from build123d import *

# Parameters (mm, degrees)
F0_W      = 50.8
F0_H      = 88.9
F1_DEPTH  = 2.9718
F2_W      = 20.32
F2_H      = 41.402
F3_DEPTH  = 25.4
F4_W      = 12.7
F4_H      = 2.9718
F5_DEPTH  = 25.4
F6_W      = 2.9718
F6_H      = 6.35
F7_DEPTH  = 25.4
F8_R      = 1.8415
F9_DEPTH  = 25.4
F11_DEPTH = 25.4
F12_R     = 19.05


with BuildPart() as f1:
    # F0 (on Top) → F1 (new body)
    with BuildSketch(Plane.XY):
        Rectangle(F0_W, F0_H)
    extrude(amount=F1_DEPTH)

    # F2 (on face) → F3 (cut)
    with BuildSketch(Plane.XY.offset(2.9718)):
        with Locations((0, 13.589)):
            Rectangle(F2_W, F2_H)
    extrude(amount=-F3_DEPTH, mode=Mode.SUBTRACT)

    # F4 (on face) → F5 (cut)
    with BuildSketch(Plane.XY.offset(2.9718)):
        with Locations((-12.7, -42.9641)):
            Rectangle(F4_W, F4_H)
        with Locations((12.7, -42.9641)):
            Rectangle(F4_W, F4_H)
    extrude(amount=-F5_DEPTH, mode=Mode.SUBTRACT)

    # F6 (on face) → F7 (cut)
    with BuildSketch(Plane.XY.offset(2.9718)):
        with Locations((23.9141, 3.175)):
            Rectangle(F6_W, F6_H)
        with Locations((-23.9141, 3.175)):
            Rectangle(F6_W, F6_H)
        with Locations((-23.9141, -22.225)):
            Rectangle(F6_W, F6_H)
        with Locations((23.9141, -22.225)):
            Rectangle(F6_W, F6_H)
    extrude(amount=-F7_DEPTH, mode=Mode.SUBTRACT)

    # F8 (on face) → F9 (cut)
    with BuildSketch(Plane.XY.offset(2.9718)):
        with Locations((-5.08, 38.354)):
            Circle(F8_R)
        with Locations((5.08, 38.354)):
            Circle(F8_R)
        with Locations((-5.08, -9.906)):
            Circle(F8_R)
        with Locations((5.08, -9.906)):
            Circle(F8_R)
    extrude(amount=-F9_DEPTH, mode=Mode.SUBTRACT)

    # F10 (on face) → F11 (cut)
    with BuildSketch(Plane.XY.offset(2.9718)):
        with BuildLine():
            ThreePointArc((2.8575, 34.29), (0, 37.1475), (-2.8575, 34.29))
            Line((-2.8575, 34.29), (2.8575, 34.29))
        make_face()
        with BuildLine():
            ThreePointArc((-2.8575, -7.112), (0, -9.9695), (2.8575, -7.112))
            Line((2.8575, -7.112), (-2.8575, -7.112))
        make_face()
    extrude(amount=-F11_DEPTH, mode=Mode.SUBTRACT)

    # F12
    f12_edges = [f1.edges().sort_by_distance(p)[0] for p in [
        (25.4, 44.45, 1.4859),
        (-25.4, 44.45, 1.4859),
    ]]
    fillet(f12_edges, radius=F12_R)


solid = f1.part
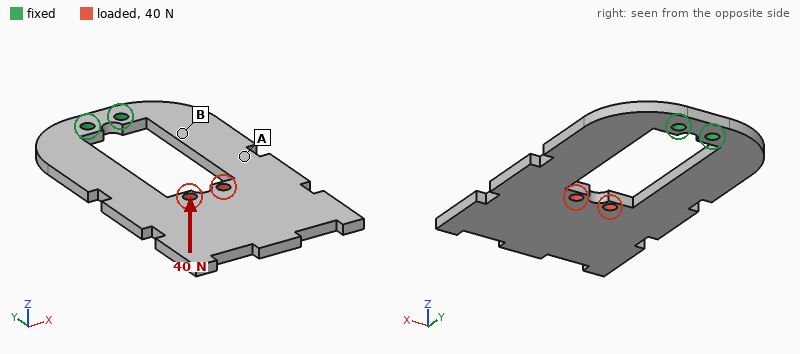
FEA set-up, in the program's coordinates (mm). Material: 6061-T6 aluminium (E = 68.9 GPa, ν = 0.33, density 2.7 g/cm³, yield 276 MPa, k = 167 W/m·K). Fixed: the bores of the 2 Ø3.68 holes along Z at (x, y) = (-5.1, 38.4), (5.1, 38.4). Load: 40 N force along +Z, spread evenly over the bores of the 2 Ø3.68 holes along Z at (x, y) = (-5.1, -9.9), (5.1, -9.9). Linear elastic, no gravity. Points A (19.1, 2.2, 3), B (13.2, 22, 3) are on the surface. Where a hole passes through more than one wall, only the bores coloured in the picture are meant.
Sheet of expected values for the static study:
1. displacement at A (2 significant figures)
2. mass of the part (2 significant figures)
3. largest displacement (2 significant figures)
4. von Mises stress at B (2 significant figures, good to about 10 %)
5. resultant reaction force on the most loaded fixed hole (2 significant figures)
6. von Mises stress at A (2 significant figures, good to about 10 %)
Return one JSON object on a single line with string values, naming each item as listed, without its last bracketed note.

{"displacement at A": "0.35 mm", "mass of the part": "26 g", "largest displacement": "1.0 mm", "von Mises stress at B": "30 MPa", "resultant reaction force on the most loaded fixed hole": "20 N", "von Mises stress at A": "14 MPa"}
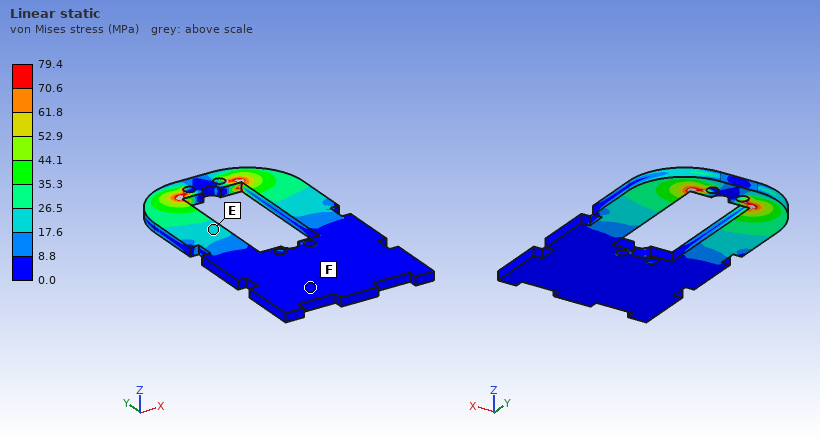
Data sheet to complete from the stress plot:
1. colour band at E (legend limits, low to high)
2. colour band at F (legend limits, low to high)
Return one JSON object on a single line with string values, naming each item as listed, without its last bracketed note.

{"colour band at E": "17.6 to 26.5 MPa", "colour band at F": "0.0 to 8.8 MPa"}
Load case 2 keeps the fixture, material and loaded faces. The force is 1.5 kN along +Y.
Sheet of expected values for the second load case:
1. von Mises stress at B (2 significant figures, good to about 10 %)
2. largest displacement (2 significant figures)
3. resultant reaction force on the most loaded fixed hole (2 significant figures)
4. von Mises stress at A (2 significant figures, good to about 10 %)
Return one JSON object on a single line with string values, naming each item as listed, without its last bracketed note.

{"von Mises stress at B": "35 MPa", "largest displacement": "46 µm", "resultant reaction force on the most loaded fixed hole": "800 N", "von Mises stress at A": "16 MPa"}
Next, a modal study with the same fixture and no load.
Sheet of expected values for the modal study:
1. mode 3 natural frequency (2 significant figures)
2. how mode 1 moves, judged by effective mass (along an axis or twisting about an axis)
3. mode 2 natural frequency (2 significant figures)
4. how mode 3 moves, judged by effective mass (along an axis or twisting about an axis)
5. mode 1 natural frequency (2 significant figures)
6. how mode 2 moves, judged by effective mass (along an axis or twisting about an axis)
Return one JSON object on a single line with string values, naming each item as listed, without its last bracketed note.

{"mode 3 natural frequency": "1200 Hz", "how mode 1 moves, judged by effective mass": "along Z", "mode 2 natural frequency": "830 Hz", "how mode 3 moves, judged by effective mass": "along X", "mode 1 natural frequency": "240 Hz", "how mode 2 moves, judged by effective mass": "twisting about Y"}
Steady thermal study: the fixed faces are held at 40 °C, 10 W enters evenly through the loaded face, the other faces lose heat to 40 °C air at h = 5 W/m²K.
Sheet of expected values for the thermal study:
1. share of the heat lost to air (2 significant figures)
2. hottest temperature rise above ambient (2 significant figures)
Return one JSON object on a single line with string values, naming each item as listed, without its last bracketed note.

{"share of the heat lost to air": "12 %", "hottest temperature rise above ambient": "48 K"}
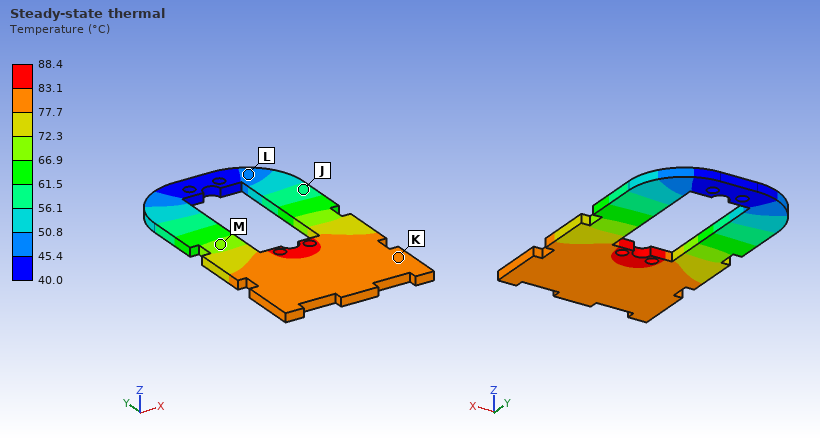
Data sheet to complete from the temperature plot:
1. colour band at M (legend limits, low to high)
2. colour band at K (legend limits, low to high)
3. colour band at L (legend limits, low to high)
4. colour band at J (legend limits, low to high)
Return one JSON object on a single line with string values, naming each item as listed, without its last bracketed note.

{"colour band at M": "66.9 to 72.3 °C", "colour band at K": "77.7 to 83.1 °C", "colour band at L": "45.4 to 50.8 °C", "colour band at J": "56.1 to 61.5 °C"}
